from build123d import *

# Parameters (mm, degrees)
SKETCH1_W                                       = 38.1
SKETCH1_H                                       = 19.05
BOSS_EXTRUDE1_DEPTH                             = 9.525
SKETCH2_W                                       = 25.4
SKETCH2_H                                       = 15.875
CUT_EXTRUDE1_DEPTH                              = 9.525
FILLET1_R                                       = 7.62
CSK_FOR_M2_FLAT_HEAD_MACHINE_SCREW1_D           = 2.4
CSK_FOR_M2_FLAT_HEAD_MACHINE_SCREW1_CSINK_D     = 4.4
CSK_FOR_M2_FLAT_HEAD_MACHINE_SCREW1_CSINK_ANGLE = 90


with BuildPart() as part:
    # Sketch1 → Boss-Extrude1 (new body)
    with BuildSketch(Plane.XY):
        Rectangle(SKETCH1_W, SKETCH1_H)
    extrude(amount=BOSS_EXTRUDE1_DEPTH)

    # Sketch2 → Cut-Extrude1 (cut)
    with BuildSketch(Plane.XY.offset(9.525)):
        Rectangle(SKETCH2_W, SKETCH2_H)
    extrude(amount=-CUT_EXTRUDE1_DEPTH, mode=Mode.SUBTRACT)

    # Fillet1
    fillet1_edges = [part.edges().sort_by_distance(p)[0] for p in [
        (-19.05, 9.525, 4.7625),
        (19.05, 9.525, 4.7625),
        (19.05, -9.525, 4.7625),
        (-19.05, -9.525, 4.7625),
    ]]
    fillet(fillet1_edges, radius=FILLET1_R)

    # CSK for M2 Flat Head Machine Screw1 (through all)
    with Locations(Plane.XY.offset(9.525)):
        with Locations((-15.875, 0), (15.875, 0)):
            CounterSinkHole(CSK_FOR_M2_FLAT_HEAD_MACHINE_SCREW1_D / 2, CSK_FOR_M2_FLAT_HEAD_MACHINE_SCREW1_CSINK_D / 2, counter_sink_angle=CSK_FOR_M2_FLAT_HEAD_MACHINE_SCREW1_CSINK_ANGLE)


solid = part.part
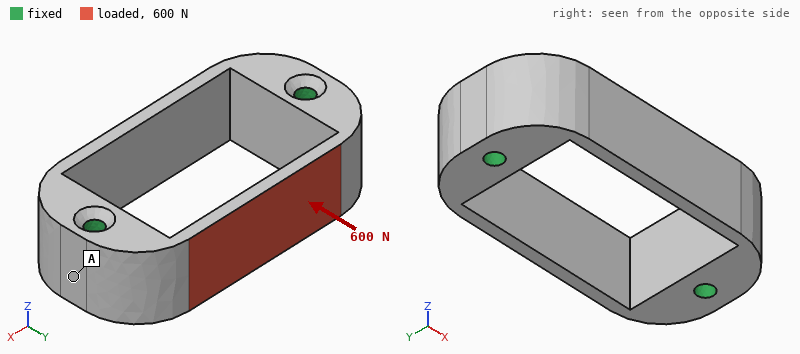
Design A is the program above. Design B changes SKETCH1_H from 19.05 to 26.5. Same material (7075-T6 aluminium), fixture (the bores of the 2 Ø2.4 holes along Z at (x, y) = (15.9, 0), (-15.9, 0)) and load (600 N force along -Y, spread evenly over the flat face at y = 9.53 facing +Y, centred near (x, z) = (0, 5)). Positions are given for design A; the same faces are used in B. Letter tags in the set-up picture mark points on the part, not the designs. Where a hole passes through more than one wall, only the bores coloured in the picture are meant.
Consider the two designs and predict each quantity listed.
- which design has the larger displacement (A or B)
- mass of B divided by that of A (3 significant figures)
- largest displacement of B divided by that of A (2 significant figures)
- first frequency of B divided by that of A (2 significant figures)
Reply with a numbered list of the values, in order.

1. A
2. 2.08
3. 0.064
4. 1.5
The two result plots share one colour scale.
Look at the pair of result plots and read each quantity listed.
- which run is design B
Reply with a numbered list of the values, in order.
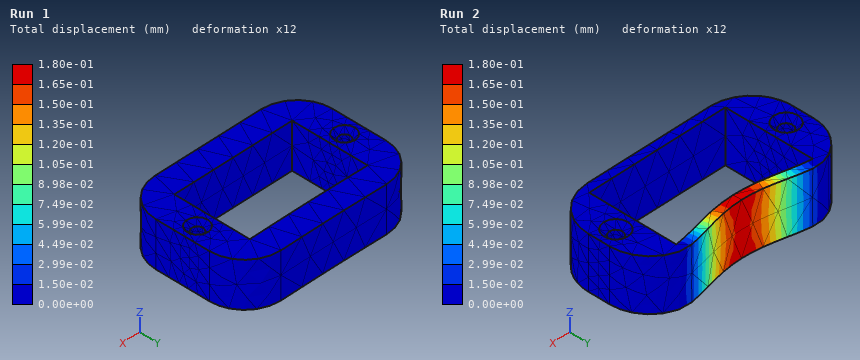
1. Run 1
